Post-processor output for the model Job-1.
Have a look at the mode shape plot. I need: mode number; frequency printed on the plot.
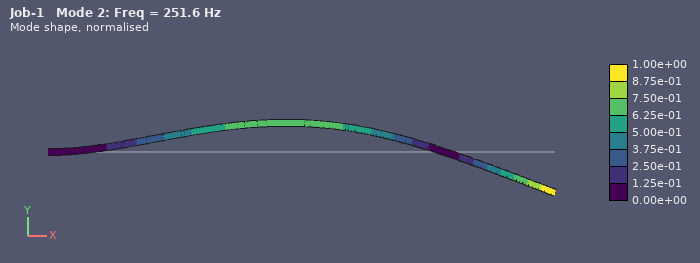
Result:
2
251.6 Hz
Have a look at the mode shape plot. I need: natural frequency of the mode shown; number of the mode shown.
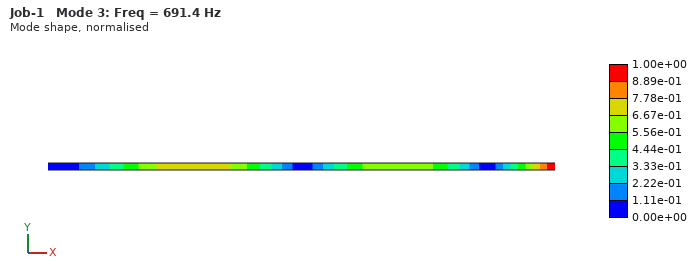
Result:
691.4 Hz
3
